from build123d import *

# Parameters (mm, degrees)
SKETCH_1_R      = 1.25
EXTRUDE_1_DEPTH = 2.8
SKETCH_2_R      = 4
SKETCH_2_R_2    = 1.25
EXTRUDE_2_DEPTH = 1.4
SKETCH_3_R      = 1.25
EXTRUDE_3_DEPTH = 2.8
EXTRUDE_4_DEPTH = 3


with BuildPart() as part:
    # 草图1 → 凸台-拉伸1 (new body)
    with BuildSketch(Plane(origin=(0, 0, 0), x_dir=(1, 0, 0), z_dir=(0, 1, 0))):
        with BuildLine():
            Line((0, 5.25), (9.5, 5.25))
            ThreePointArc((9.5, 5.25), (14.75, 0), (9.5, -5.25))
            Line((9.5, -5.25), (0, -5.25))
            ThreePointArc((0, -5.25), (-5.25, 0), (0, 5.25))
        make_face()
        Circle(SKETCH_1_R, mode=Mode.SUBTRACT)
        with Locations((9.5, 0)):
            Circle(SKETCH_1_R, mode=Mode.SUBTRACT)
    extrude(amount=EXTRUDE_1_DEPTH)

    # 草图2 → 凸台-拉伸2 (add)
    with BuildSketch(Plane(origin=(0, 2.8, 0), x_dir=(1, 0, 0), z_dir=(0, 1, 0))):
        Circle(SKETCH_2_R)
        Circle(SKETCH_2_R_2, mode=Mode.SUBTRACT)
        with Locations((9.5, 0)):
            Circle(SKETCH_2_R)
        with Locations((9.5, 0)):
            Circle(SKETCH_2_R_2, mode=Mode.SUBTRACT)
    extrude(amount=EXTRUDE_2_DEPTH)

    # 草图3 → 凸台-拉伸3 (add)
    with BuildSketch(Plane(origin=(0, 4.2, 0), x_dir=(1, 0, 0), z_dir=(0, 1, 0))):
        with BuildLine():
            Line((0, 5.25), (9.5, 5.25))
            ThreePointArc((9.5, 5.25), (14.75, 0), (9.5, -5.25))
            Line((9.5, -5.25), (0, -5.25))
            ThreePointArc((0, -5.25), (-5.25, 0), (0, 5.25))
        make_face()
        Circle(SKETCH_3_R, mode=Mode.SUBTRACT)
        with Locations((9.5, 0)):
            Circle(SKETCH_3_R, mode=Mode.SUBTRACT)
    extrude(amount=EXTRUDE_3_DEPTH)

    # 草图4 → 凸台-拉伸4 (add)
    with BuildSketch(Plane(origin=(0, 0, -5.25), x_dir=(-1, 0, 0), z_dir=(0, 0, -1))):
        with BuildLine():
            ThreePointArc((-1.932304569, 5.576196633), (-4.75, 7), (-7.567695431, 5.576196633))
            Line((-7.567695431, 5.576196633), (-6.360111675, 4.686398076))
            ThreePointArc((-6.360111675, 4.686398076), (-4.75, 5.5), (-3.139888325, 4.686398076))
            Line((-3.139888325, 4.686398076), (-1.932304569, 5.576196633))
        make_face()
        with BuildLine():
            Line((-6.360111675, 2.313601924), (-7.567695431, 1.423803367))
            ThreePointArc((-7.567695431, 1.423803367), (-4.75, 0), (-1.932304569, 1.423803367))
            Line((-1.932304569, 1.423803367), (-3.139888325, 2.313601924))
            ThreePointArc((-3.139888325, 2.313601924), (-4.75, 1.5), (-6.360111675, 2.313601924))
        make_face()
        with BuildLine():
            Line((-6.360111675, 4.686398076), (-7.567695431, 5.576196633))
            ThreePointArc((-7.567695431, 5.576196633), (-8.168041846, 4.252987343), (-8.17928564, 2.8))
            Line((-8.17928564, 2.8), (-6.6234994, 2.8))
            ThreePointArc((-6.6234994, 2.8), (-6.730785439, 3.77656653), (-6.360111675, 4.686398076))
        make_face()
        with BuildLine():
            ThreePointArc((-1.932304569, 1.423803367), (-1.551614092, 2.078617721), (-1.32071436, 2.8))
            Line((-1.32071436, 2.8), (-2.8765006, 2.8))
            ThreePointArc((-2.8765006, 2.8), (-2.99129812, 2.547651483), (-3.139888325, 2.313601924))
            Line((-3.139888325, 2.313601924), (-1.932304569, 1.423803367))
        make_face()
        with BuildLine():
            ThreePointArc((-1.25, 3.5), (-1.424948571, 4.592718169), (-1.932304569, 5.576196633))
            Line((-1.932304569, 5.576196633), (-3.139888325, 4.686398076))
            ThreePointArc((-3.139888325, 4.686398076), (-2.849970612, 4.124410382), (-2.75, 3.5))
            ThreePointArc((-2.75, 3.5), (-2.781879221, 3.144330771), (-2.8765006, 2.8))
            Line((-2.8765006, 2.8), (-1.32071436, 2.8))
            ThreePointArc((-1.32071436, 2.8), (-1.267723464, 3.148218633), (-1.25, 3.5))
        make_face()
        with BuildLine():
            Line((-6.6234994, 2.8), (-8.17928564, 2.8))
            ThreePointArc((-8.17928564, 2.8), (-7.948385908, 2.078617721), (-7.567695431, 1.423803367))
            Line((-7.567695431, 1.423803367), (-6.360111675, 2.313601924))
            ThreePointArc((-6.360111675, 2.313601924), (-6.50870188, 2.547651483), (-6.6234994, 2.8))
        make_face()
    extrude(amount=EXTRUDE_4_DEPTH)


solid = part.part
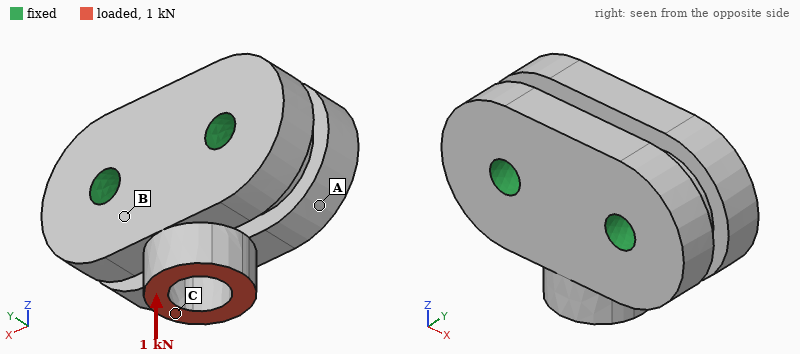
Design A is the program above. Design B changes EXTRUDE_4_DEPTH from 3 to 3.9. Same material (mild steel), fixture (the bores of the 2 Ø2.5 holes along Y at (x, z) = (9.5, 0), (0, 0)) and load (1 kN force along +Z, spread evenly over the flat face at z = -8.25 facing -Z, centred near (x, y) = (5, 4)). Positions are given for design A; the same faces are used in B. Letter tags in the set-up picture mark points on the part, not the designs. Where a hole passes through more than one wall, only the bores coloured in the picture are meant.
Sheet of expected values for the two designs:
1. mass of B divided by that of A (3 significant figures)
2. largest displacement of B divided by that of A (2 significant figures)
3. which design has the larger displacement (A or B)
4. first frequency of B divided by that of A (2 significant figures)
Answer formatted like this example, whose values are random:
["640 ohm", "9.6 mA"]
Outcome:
["1.02", "1.1", "B", "0.87"]
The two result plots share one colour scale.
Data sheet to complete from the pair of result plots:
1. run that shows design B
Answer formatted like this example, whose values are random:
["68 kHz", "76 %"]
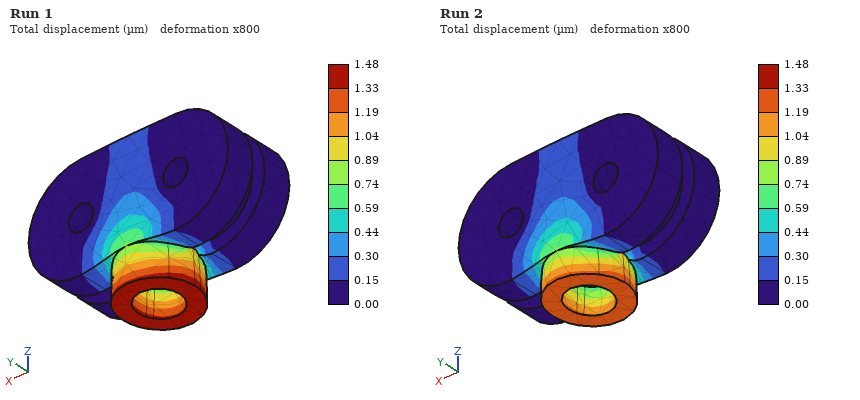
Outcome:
["Run 1"]
